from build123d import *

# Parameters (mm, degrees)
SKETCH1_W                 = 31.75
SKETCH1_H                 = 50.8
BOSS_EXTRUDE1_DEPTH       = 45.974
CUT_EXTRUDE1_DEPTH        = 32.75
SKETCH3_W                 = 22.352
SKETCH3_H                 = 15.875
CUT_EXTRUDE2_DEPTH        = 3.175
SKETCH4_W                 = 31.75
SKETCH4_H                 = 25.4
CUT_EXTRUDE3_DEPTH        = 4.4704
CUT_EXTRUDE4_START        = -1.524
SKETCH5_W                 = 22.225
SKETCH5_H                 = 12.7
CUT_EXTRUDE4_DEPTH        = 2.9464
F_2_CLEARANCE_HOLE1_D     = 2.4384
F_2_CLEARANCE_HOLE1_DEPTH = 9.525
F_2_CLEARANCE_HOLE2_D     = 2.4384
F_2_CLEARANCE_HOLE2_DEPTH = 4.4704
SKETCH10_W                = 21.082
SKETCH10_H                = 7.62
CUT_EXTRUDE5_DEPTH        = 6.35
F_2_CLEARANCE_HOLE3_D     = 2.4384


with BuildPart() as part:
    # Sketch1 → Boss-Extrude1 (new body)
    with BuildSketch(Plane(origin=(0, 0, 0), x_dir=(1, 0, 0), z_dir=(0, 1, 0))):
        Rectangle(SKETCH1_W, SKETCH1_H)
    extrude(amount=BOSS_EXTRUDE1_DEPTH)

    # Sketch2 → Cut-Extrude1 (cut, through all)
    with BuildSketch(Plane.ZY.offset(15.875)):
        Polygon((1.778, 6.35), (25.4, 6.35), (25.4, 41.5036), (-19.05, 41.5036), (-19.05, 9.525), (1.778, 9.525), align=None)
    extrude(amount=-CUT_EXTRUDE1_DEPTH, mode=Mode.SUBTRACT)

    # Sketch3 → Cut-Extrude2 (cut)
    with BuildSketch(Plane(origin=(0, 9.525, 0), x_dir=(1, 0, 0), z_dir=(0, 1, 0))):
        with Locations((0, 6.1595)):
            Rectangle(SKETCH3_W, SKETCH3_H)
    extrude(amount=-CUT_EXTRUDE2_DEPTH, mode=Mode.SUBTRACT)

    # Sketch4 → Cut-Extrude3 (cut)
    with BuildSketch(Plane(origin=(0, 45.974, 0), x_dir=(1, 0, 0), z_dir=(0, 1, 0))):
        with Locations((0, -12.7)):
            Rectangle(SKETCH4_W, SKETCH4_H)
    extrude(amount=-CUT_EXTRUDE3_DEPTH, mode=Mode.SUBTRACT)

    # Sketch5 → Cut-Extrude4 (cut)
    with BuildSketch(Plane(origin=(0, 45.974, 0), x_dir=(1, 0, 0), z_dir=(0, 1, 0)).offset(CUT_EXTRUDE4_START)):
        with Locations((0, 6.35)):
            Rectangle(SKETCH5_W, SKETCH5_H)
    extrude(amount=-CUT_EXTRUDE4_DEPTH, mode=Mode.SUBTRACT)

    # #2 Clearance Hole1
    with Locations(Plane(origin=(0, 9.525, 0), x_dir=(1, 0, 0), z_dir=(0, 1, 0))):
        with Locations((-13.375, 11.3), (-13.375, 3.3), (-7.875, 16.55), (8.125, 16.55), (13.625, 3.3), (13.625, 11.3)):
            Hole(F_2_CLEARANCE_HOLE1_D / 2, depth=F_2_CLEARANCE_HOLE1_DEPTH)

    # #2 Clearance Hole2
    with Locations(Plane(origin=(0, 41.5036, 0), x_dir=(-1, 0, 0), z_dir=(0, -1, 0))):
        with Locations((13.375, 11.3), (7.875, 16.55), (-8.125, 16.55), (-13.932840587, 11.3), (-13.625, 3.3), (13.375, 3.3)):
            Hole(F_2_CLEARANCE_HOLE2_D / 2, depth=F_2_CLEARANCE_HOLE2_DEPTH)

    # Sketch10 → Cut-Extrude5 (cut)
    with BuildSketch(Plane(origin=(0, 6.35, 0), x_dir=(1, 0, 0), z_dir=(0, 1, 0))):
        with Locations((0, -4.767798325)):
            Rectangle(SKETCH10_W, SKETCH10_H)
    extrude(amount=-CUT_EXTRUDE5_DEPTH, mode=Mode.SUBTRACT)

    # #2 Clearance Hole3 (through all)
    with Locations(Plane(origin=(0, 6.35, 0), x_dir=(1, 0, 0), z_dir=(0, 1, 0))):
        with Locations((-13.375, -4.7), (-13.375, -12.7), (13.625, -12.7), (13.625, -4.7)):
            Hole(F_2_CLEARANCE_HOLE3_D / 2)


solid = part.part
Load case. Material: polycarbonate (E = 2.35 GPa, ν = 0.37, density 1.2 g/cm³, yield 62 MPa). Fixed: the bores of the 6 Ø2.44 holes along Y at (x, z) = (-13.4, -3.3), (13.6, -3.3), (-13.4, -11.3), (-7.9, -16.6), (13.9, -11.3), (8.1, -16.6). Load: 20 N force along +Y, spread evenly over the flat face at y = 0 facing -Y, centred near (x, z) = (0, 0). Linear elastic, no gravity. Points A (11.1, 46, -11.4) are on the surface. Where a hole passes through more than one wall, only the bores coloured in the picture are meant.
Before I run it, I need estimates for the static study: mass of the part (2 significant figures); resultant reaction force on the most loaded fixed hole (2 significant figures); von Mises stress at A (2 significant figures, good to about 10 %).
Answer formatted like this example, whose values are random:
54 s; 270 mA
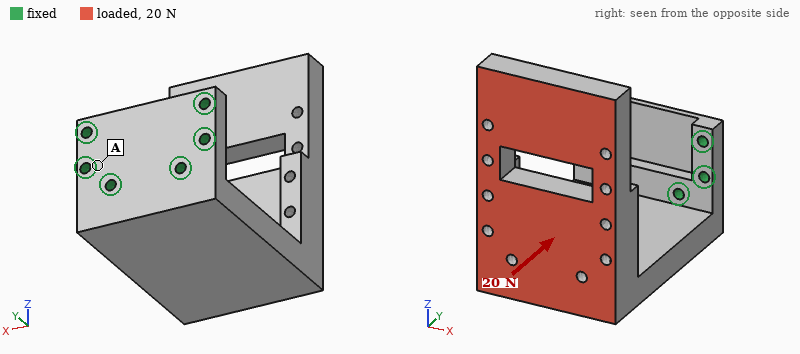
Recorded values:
23 g; 7.7 N; 0.47 MPa
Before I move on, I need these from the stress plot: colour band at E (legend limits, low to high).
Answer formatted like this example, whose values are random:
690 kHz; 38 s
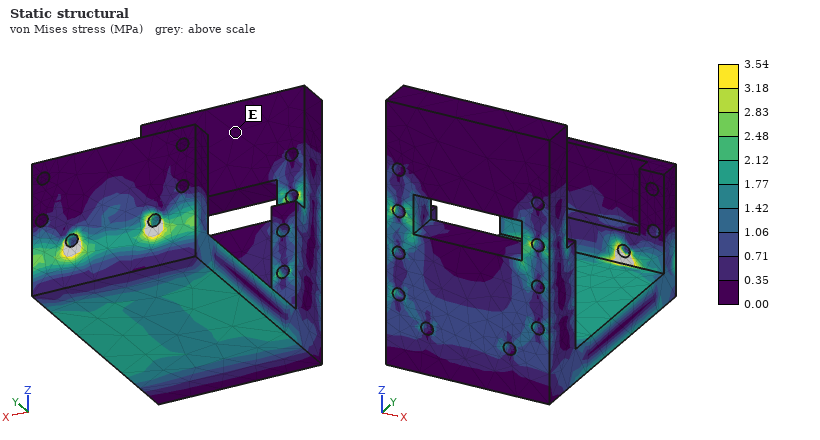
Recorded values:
0.00 to 0.35 MPa
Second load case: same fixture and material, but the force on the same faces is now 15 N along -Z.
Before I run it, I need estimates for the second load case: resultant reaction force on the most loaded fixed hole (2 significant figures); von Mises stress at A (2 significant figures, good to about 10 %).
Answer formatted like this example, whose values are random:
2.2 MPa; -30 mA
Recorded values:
17 N; 0.86 MPa
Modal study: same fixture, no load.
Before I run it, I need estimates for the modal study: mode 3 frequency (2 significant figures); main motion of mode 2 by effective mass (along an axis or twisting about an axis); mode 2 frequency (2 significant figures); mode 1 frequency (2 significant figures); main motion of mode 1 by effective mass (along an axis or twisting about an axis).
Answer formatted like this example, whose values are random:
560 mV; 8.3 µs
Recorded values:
630 Hz; along X; 370 Hz; 210 Hz; along Z
